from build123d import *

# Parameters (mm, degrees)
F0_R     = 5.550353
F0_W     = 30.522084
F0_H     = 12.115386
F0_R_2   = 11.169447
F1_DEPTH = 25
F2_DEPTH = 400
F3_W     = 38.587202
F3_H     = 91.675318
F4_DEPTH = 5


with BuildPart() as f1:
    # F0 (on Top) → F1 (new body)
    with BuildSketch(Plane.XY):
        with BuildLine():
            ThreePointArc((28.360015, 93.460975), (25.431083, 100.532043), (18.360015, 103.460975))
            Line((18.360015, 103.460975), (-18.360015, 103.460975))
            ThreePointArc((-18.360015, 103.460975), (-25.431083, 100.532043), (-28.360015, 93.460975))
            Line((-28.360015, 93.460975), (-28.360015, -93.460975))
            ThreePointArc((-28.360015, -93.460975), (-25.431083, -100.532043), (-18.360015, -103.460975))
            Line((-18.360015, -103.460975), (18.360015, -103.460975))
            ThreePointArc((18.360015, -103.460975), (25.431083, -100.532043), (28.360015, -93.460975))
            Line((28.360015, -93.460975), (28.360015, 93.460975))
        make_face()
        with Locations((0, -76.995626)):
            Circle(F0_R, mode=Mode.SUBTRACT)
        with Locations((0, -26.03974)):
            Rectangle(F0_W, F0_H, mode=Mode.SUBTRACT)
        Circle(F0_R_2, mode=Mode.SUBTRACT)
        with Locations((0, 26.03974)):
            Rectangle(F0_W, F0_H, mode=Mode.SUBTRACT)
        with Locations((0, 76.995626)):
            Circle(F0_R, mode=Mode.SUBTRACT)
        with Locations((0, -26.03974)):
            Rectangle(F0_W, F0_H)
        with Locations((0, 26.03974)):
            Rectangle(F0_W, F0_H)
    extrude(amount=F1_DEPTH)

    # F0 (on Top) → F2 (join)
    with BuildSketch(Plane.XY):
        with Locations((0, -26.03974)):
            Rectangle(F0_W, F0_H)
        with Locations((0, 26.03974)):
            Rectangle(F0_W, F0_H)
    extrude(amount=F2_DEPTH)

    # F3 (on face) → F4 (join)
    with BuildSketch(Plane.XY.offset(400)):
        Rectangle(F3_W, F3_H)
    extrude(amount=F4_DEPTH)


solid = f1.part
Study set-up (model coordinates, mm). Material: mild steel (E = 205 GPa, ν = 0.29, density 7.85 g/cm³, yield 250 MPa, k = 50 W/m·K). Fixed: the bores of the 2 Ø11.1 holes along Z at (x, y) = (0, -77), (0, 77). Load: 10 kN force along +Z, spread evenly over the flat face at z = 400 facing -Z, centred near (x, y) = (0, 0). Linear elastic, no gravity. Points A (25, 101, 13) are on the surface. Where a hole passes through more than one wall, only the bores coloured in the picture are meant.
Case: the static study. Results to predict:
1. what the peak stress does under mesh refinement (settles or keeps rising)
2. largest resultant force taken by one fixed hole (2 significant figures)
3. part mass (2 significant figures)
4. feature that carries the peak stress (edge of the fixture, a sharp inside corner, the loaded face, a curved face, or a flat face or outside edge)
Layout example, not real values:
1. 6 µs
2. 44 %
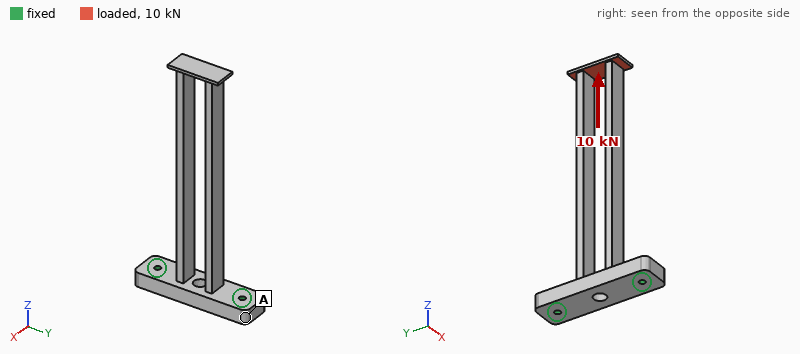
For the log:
1. keeps rising
2. 5.0 kN
3. 4.5 kg
4. edge of the fixture
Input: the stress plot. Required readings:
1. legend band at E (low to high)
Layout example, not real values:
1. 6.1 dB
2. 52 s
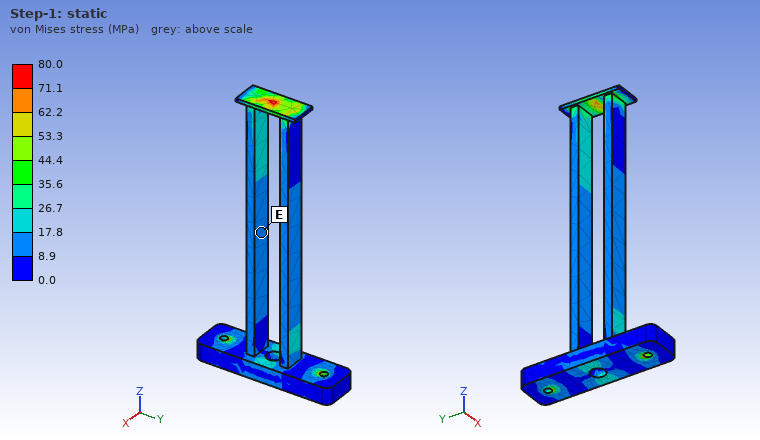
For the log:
1. 8.9 to 17.8 MPa
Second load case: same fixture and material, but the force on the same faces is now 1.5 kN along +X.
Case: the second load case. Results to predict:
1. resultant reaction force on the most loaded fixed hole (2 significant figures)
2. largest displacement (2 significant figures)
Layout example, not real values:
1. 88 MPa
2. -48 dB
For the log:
1. 750 N
2. 2.7 mm
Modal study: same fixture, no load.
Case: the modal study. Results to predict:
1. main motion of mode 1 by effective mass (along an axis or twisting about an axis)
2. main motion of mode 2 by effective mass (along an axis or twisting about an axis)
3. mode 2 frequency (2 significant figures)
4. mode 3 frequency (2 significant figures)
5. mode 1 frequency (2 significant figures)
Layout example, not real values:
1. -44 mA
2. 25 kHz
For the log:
1. along Y
2. along X
3. 140 Hz
4. 330 Hz
5. 93 Hz
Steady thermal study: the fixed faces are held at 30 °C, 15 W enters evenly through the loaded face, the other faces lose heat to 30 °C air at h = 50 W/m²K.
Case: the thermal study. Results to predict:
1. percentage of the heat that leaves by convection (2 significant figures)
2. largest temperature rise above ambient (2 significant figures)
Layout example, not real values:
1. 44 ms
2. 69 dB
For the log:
1. 100 %
2. 22 K
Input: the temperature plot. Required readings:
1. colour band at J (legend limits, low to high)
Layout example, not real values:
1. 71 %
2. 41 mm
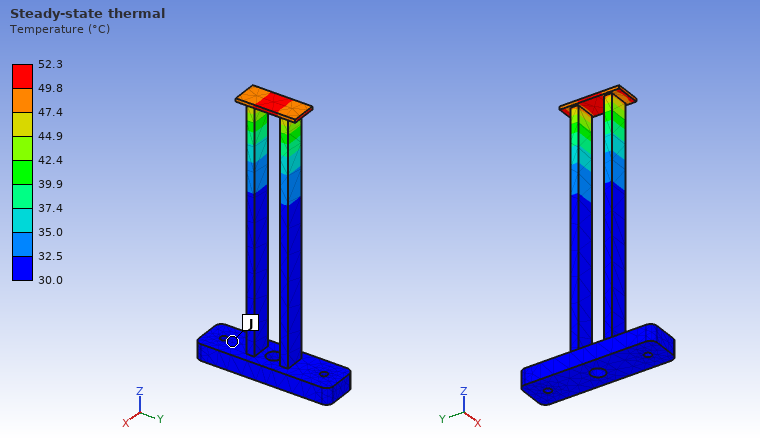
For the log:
1. 30.0 to 32.5 °C
